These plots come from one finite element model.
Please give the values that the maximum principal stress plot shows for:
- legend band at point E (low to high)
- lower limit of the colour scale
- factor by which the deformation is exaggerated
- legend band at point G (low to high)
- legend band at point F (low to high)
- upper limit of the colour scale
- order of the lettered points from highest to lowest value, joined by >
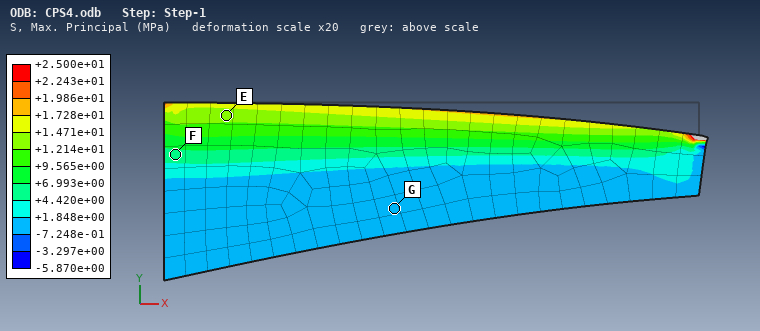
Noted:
+1.214e+01 to +1.471e+01 MPa
-5.870e+00 MPa
20
-7.248e-01 to +1.848e+00 MPa
+4.420e+00 to +6.993e+00 MPa
+2.500e+01 MPa
E > F > G
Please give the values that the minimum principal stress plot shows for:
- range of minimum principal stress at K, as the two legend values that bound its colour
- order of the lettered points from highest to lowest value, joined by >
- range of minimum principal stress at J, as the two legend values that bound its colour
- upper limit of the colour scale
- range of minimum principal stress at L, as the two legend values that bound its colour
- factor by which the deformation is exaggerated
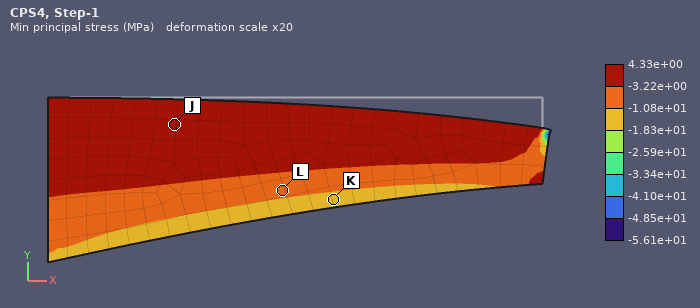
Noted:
-1.83e+01 to -1.08e+01 MPa
J > L > K
-3.22e+00 to 4.33e+00 MPa
4.33e+00 MPa
-1.08e+01 to -3.22e+00 MPa
20
